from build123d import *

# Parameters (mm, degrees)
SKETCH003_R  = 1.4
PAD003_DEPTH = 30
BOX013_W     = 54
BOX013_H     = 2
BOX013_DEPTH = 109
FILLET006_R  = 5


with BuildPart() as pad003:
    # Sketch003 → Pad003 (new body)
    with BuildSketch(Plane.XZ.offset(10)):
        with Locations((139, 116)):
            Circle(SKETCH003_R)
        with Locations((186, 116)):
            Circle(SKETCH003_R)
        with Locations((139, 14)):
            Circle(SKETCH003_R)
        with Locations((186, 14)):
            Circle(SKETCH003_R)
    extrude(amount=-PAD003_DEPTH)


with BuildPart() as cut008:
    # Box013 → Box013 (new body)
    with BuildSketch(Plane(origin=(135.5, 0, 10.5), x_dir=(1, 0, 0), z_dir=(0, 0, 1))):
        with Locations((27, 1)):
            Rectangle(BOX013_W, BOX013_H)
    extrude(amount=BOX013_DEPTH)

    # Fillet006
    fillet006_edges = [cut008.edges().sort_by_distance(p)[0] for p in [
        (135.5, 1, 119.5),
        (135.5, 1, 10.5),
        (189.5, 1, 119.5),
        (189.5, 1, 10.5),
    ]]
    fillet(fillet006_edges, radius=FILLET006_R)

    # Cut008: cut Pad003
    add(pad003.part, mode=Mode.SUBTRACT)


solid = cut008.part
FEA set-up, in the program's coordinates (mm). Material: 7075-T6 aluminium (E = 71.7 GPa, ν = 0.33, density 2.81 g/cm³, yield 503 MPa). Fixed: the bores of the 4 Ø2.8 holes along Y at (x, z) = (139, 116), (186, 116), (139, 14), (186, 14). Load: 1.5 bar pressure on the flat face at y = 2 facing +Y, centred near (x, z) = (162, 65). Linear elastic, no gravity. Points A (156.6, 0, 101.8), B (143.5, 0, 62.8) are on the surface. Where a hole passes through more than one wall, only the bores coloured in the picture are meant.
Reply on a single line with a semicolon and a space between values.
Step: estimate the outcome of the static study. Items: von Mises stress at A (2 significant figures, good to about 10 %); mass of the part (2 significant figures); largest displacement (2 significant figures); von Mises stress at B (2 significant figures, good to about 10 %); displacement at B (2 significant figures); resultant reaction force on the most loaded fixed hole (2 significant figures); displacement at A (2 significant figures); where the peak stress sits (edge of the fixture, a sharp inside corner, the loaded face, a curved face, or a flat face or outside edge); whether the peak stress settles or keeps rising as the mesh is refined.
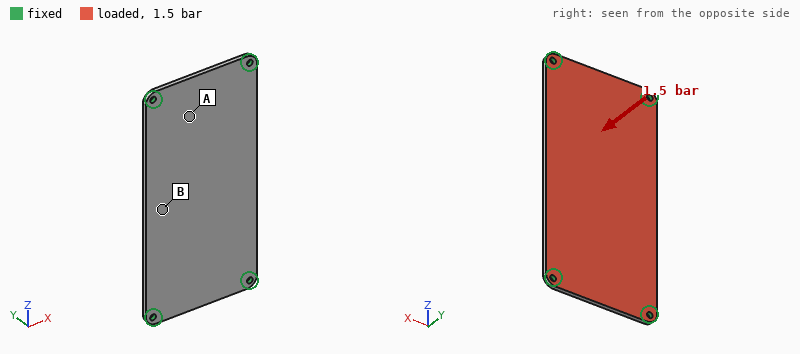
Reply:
41 MPa; 33 g; 1.2 mm; 110 MPa; 1.2 mm; 220 N; 0.43 mm; edge of the fixture; keeps rising
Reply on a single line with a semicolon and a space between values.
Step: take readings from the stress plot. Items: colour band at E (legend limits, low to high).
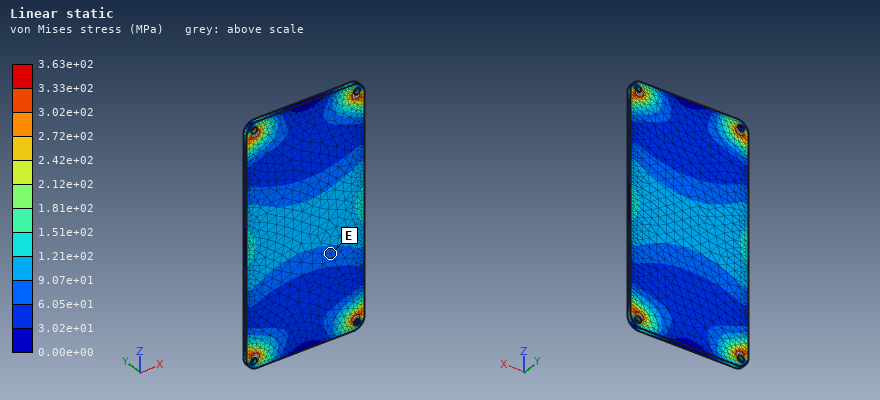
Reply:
6.05e+01 to 9.07e+01 MPa
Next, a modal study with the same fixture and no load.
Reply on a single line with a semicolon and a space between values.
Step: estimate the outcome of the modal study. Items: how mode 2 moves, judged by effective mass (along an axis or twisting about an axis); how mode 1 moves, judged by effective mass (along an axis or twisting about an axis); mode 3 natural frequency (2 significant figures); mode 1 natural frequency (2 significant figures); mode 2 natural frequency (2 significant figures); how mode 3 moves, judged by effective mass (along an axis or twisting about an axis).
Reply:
twisting about Z; along Y; 2400 Hz; 850 Hz; 1600 Hz; twisting about X
